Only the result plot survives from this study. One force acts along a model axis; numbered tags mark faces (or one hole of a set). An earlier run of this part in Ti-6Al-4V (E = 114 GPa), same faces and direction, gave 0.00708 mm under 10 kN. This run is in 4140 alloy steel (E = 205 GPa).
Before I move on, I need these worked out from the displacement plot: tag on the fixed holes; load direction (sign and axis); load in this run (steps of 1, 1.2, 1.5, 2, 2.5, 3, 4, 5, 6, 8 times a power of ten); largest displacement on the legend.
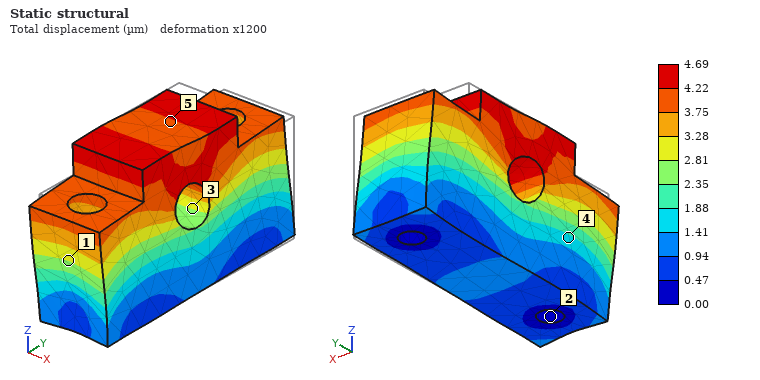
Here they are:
2
-Y
12 kN
4.69 µm
